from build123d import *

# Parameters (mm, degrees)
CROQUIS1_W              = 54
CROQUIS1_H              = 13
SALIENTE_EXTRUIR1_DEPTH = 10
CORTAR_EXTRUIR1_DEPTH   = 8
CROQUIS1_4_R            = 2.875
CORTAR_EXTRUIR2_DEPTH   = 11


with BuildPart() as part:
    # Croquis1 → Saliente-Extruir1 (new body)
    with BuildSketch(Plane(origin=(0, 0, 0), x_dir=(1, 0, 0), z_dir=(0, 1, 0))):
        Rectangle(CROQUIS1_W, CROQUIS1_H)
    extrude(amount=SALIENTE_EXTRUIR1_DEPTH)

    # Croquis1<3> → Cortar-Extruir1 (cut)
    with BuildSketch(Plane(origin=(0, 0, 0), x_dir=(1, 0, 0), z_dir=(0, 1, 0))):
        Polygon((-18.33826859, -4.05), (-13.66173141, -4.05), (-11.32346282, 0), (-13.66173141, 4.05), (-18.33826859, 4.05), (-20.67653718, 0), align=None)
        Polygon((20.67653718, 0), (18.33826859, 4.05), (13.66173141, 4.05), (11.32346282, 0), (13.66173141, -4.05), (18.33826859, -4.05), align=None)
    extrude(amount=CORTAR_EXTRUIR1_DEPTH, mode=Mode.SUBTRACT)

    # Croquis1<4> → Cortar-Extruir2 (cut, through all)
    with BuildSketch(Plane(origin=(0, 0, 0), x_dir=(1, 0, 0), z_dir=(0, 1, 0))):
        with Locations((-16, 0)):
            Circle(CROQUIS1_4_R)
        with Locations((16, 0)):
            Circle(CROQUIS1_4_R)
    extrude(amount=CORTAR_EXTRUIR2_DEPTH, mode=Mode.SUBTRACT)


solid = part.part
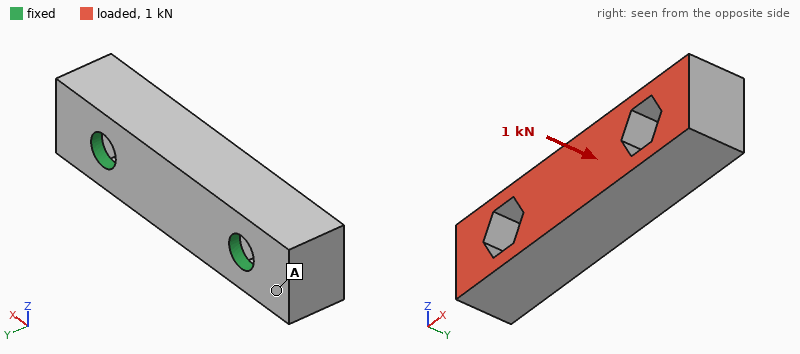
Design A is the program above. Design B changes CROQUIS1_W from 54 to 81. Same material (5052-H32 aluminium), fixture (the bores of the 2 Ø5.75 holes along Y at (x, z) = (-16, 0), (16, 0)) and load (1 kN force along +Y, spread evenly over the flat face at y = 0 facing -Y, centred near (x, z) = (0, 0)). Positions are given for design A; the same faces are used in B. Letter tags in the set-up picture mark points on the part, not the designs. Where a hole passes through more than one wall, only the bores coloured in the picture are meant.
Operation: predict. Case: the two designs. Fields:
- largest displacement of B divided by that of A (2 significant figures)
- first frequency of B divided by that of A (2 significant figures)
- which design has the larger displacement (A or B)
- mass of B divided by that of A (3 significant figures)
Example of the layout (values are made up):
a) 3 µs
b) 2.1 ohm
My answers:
a) 6.8
b) 0.60
c) B
d) 1.58
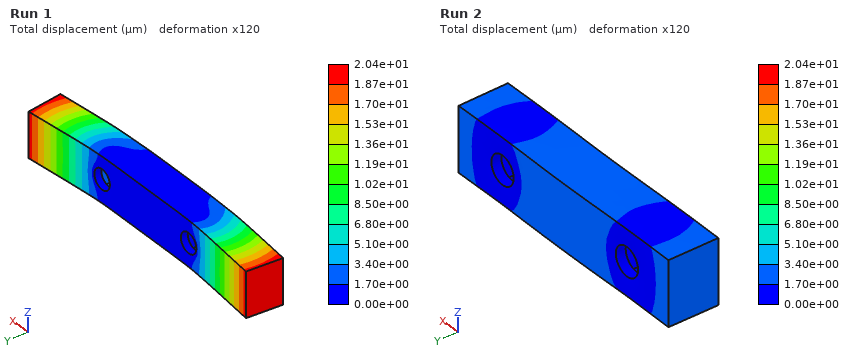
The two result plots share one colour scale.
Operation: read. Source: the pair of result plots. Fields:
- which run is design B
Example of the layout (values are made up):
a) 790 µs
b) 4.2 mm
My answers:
a) Run 1
